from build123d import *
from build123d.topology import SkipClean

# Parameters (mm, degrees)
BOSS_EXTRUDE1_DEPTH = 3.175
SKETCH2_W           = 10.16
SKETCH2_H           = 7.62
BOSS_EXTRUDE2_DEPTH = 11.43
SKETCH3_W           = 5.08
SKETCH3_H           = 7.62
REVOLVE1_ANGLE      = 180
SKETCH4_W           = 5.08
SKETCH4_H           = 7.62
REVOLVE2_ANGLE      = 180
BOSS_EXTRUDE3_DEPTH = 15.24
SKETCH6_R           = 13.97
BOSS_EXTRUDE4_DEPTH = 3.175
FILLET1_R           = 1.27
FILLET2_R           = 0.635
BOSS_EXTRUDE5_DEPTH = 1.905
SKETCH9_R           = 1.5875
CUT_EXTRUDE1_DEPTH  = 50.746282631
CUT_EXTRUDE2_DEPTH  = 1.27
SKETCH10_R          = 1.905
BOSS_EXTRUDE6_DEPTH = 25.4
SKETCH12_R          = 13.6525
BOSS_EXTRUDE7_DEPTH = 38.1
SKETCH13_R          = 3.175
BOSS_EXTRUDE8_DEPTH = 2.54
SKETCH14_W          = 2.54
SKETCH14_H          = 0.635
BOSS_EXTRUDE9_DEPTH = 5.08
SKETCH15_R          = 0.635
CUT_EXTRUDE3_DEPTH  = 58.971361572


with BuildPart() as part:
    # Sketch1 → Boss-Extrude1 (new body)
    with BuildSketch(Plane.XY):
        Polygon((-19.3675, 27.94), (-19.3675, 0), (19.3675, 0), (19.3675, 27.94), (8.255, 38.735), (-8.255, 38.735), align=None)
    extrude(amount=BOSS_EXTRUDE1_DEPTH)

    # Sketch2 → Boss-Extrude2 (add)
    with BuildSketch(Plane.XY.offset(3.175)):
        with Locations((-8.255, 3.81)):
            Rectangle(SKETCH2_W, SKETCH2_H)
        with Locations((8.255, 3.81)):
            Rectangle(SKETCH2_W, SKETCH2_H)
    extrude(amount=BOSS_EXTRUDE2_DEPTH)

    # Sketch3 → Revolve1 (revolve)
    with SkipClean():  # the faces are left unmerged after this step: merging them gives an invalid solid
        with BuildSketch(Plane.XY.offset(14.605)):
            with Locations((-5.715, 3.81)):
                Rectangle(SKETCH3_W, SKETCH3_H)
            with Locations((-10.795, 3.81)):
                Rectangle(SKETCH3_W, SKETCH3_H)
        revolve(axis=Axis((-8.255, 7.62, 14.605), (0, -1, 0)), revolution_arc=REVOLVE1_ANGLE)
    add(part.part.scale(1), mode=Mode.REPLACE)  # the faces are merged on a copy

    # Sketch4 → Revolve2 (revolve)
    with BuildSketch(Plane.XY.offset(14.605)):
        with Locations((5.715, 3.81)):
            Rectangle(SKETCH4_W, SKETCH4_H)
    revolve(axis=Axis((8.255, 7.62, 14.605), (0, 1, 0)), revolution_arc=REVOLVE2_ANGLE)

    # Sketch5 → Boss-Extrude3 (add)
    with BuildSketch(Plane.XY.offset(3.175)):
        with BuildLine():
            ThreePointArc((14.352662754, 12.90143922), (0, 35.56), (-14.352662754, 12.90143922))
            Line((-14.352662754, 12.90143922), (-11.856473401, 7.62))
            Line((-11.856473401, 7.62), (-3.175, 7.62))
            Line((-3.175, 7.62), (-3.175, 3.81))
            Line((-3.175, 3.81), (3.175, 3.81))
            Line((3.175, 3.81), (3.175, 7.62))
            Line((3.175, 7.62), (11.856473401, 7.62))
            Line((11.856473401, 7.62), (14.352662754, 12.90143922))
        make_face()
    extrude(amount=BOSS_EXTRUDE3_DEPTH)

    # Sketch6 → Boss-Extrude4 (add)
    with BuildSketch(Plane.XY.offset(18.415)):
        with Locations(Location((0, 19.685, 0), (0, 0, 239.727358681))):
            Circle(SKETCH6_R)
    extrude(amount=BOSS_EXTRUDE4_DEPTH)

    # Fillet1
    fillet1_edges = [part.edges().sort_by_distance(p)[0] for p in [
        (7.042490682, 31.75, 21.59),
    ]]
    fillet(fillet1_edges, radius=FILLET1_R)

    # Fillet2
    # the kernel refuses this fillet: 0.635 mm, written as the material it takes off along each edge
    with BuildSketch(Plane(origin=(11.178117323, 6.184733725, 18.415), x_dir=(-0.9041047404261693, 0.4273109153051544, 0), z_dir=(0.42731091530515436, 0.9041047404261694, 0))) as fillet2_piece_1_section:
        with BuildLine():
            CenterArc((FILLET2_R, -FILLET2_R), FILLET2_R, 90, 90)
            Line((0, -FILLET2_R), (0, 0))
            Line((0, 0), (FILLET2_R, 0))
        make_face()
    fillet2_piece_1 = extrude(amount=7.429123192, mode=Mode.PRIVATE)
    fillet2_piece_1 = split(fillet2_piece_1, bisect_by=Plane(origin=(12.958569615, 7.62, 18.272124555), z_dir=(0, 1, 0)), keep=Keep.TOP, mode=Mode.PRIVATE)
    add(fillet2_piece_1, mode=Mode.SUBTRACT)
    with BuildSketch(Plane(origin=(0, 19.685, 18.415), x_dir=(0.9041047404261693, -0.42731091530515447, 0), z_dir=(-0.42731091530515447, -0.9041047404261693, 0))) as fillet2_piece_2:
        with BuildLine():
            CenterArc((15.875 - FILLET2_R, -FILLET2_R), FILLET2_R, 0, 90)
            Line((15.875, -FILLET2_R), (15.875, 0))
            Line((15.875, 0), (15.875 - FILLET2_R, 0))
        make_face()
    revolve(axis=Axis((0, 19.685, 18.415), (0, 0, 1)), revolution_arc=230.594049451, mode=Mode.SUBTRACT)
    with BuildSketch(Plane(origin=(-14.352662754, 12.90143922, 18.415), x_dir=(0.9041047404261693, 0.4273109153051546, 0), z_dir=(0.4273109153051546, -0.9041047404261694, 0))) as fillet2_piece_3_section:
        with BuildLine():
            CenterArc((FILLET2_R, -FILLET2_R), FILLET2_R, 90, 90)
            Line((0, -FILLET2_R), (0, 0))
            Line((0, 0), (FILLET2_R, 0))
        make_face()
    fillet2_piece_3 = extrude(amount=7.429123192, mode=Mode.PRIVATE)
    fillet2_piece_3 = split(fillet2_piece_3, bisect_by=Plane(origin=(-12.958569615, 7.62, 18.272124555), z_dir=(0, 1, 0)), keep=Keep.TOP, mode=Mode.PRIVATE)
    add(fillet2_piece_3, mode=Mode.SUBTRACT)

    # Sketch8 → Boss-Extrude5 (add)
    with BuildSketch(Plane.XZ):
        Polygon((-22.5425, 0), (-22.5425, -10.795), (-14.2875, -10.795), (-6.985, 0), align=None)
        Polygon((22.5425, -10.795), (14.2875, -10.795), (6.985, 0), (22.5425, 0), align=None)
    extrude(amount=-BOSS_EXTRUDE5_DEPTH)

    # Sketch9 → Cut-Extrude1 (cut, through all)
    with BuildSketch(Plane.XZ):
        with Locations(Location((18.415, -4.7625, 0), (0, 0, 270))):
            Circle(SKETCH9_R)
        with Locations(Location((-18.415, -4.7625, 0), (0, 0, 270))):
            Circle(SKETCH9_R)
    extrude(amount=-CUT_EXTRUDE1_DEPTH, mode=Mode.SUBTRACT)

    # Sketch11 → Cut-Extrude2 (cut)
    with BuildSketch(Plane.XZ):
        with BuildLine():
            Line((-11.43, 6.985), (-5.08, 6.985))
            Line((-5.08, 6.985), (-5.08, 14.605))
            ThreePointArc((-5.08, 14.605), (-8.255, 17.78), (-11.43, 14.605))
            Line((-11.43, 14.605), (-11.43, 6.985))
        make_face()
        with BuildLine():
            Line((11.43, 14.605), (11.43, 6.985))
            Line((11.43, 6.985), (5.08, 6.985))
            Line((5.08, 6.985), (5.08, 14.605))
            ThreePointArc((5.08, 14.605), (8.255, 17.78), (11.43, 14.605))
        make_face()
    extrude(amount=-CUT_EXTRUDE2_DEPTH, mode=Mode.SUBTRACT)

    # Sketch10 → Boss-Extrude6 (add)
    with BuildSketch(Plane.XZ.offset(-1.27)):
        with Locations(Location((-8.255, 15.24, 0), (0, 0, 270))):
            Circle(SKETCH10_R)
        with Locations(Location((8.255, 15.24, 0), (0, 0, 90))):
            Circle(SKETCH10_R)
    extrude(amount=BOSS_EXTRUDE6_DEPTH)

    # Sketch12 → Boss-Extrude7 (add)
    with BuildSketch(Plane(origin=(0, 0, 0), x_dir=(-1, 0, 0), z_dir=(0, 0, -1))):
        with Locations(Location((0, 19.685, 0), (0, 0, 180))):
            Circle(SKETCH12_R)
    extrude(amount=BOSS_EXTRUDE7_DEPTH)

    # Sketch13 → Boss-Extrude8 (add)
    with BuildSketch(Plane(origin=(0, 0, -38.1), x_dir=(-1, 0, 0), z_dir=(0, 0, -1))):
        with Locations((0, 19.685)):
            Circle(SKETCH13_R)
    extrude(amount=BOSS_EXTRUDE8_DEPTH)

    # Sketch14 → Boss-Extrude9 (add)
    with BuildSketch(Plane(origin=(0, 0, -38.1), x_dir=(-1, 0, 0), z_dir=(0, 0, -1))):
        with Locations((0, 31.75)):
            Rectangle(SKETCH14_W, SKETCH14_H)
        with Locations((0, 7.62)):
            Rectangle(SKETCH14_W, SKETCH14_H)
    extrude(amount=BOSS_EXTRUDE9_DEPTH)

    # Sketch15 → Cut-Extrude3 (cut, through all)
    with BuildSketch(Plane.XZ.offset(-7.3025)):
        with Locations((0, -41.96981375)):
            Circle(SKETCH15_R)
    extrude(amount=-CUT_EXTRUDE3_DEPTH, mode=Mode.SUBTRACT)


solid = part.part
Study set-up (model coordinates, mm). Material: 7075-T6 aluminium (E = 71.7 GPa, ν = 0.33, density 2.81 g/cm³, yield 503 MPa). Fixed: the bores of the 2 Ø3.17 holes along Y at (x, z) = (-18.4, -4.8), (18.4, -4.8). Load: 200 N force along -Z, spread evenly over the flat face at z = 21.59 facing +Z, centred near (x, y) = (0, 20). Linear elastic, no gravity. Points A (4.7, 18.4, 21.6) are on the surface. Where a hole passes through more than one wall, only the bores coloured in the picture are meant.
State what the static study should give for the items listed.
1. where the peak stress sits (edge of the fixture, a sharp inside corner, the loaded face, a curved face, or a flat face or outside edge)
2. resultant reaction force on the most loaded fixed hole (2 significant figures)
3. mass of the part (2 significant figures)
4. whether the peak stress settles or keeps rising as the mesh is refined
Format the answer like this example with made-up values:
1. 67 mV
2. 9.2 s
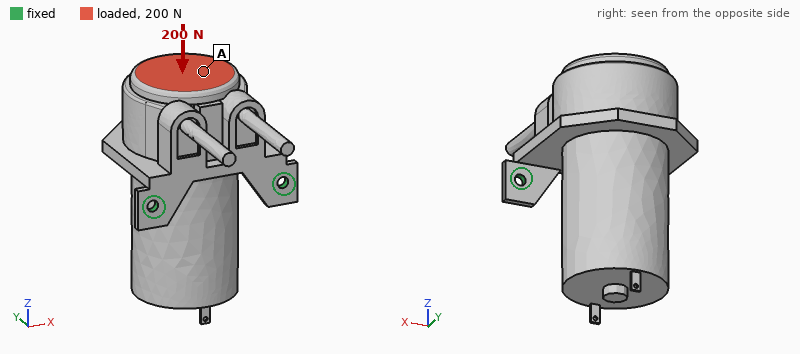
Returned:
1. edge of the fixture
2. 100 N
3. 120 g
4. keeps rising
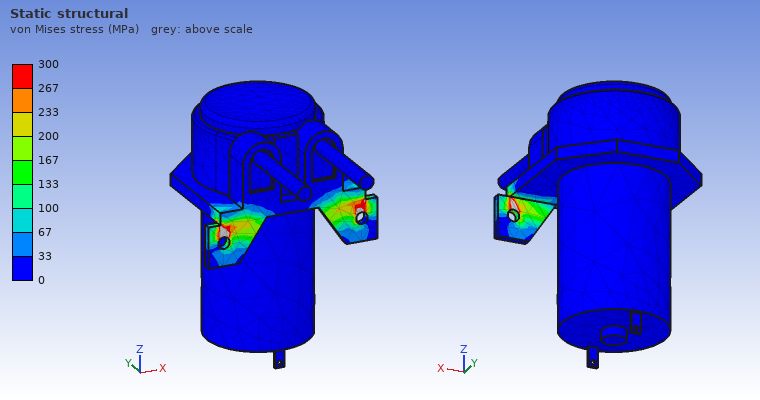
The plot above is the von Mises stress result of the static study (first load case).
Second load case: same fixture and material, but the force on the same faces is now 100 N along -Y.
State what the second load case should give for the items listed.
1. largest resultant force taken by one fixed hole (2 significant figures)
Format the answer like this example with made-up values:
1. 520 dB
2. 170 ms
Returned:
1. 67 N
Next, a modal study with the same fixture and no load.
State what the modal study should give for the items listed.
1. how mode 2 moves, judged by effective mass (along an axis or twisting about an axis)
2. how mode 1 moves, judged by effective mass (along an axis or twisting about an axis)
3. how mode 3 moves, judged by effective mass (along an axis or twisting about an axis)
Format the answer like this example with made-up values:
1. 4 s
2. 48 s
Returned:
1. along X
2. along Z
3. along Y
